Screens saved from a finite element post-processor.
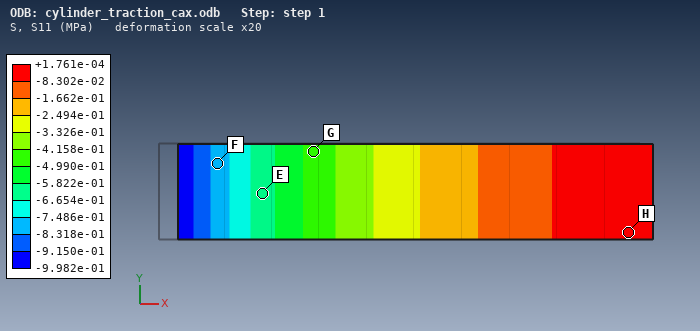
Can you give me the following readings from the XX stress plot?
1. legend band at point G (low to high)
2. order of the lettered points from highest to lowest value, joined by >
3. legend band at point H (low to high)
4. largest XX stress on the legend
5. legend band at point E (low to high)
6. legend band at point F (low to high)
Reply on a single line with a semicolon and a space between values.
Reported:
-4.990e-01 to -4.158e-01 MPa; H > G > E > F; -8.302e-02 to +1.761e-04 MPa; +1.761e-04 MPa; -6.654e-01 to -5.822e-01 MPa; -8.318e-01 to -7.486e-01 MPa
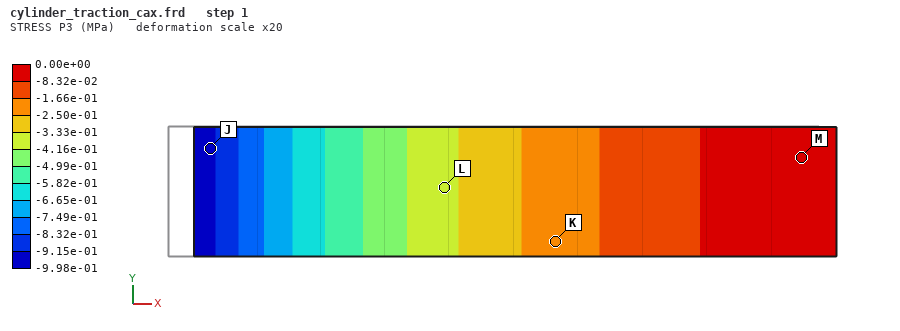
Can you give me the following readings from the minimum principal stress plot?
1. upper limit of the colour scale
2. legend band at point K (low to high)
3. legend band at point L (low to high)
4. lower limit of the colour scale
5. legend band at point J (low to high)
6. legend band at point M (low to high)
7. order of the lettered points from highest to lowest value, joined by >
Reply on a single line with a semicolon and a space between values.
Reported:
0.00e+00 MPa; -2.50e-01 to -1.66e-01 MPa; -4.16e-01 to -3.33e-01 MPa; -9.98e-01 MPa; -9.98e-01 to -9.15e-01 MPa; -8.32e-02 to 0.00e+00 MPa; M > K > L > J
